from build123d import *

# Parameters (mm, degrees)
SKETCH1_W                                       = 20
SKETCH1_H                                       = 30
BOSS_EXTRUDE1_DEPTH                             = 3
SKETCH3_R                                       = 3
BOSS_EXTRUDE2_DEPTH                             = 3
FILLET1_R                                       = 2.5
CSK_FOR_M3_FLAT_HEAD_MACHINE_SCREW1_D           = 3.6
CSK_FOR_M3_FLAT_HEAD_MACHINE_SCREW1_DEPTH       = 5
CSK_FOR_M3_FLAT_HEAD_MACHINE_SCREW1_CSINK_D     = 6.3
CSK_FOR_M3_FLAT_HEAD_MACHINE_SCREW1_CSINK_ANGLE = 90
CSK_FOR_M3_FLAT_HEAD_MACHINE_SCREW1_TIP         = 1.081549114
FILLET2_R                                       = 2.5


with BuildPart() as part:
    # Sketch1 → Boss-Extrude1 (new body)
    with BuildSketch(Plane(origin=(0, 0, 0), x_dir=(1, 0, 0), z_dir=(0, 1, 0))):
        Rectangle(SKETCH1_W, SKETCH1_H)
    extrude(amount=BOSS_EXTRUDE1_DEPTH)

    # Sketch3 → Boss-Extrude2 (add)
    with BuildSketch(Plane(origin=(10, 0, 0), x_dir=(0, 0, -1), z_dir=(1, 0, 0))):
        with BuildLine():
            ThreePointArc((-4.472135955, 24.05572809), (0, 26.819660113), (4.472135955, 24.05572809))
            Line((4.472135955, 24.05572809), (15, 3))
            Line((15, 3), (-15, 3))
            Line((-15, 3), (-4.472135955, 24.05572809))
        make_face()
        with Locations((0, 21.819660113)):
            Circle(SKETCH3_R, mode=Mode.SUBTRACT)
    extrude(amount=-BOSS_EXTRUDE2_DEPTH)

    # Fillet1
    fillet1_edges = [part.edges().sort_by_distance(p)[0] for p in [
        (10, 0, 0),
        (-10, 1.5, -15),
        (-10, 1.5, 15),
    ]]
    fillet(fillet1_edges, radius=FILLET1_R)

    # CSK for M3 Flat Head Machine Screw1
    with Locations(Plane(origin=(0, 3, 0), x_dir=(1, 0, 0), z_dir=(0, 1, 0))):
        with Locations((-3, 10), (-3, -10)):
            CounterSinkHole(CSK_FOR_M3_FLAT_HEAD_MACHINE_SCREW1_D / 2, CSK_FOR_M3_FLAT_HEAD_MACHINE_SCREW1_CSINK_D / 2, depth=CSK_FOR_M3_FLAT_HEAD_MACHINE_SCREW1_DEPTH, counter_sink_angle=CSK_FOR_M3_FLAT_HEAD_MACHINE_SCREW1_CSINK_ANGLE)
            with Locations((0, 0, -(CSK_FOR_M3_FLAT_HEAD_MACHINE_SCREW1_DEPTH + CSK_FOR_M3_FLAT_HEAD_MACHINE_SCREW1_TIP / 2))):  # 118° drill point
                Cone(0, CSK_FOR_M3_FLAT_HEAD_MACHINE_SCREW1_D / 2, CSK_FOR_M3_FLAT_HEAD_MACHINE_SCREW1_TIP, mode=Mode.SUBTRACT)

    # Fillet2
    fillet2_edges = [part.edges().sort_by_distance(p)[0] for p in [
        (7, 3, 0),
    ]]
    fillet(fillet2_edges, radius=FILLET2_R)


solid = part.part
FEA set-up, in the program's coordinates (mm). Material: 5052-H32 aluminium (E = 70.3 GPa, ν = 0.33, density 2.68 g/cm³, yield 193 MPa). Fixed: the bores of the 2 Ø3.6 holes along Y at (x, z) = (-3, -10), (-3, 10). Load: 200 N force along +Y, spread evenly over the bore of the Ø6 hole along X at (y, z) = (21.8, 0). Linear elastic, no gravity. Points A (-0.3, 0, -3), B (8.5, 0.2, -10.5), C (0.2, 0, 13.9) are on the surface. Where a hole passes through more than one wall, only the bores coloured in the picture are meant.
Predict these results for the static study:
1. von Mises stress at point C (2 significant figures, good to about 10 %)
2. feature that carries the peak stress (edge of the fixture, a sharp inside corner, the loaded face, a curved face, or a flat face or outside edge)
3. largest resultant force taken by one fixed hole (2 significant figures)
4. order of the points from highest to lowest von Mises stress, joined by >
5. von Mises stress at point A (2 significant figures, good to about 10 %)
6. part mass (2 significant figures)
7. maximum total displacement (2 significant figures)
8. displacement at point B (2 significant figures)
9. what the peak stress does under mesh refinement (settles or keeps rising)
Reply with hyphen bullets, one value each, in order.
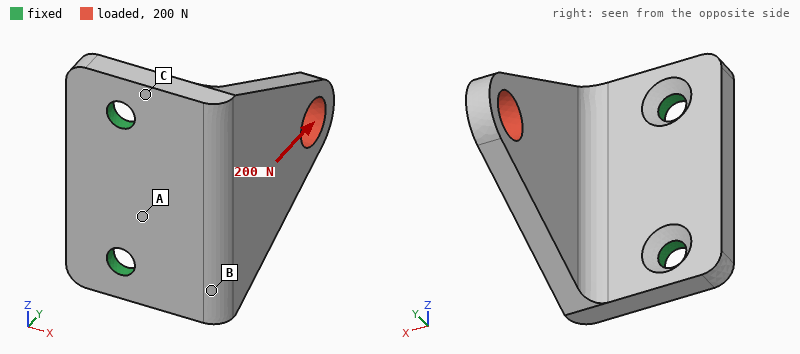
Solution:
- 43 MPa
- edge of the fixture
- 100 N
- C > A > B
- 24 MPa
- 7.8 g
- 0.10 mm
- 0.033 mm
- keeps rising
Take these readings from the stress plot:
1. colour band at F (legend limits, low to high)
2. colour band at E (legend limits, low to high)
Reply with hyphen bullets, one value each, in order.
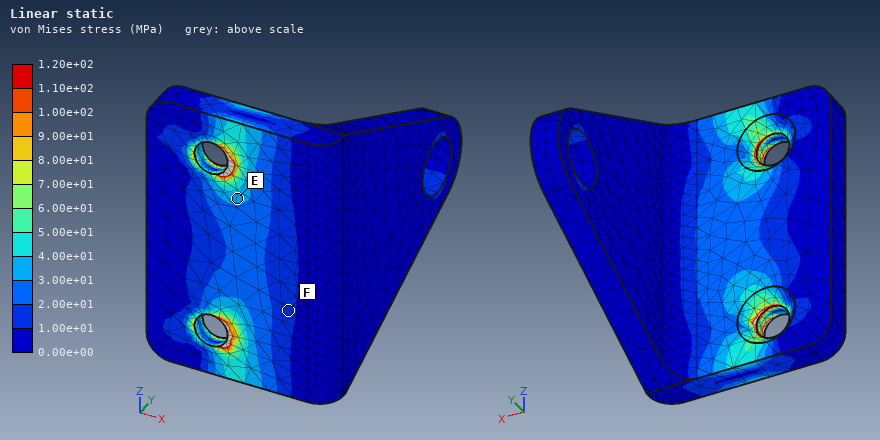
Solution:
- 1.00e+01 to 2.00e+01 MPa
- 3.00e+01 to 4.00e+01 MPa
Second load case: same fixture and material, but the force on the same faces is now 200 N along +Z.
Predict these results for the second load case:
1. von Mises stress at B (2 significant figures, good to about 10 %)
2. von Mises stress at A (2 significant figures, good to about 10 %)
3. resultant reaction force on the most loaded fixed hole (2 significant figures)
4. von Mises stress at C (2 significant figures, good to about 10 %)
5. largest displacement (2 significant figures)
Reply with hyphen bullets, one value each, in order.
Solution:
- 19 MPa
- 18 MPa
- 240 N
- 34 MPa
- 65 µm
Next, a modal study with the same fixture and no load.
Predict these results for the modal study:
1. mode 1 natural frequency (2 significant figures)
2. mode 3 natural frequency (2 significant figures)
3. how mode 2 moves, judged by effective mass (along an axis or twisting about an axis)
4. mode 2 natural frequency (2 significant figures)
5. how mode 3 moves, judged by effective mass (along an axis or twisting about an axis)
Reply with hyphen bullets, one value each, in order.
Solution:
- 3600 Hz
- 10 kHz
- along Z
- 8100 Hz
- along Y
